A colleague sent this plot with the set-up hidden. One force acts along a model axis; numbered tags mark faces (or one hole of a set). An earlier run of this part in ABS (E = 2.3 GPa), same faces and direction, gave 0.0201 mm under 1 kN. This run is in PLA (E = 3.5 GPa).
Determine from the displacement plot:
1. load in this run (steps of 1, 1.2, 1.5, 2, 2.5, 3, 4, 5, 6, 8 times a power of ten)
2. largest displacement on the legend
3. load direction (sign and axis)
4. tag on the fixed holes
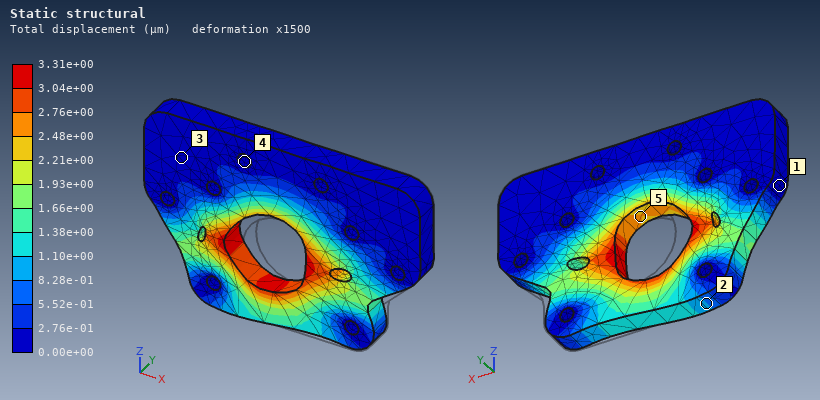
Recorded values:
250 N
3.31e+00 µm
-X
4
